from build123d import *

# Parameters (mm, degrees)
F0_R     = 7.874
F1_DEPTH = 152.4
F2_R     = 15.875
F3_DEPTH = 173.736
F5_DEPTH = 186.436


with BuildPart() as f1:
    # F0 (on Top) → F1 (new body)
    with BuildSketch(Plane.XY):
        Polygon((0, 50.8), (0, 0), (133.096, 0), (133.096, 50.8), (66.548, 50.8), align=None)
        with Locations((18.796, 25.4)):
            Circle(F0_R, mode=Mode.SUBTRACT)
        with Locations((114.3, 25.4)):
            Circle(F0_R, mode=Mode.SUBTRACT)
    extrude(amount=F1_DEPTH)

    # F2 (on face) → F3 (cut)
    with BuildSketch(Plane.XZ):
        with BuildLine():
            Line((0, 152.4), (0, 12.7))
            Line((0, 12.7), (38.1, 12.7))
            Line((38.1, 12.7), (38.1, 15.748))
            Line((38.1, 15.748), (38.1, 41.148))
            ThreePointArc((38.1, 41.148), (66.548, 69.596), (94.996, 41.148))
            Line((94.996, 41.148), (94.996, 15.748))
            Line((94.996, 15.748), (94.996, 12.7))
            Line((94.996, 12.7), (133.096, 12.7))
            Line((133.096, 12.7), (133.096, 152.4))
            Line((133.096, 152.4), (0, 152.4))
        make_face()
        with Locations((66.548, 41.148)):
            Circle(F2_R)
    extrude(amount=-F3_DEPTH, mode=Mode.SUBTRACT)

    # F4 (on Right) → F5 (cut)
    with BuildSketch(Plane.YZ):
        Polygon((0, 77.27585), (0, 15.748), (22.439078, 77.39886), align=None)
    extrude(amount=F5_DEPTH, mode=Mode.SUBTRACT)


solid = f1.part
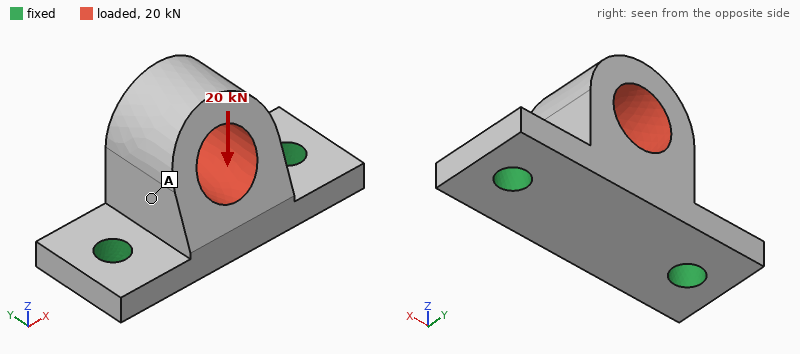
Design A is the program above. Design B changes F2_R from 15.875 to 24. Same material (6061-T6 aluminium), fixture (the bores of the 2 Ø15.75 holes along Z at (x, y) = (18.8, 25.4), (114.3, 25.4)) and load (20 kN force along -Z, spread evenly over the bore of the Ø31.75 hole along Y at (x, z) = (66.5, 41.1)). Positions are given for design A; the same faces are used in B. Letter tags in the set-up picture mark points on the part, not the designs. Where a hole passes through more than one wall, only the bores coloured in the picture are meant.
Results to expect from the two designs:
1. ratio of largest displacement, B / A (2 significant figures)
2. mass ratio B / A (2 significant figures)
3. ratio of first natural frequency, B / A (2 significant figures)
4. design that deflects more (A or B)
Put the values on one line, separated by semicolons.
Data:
2.0; 0.75; 1.3; B
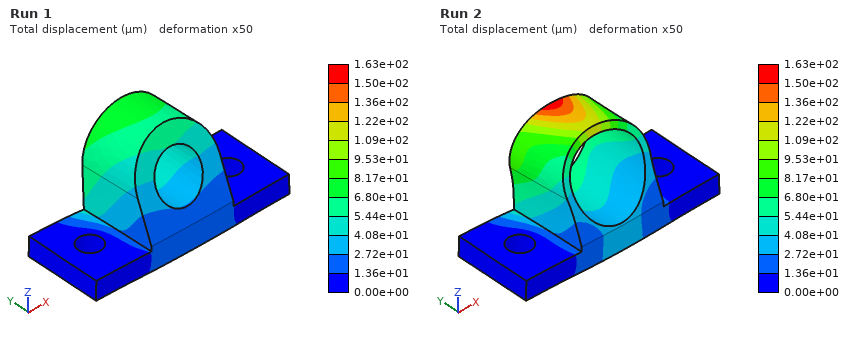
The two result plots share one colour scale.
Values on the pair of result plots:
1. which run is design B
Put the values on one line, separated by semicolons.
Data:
Run 2
